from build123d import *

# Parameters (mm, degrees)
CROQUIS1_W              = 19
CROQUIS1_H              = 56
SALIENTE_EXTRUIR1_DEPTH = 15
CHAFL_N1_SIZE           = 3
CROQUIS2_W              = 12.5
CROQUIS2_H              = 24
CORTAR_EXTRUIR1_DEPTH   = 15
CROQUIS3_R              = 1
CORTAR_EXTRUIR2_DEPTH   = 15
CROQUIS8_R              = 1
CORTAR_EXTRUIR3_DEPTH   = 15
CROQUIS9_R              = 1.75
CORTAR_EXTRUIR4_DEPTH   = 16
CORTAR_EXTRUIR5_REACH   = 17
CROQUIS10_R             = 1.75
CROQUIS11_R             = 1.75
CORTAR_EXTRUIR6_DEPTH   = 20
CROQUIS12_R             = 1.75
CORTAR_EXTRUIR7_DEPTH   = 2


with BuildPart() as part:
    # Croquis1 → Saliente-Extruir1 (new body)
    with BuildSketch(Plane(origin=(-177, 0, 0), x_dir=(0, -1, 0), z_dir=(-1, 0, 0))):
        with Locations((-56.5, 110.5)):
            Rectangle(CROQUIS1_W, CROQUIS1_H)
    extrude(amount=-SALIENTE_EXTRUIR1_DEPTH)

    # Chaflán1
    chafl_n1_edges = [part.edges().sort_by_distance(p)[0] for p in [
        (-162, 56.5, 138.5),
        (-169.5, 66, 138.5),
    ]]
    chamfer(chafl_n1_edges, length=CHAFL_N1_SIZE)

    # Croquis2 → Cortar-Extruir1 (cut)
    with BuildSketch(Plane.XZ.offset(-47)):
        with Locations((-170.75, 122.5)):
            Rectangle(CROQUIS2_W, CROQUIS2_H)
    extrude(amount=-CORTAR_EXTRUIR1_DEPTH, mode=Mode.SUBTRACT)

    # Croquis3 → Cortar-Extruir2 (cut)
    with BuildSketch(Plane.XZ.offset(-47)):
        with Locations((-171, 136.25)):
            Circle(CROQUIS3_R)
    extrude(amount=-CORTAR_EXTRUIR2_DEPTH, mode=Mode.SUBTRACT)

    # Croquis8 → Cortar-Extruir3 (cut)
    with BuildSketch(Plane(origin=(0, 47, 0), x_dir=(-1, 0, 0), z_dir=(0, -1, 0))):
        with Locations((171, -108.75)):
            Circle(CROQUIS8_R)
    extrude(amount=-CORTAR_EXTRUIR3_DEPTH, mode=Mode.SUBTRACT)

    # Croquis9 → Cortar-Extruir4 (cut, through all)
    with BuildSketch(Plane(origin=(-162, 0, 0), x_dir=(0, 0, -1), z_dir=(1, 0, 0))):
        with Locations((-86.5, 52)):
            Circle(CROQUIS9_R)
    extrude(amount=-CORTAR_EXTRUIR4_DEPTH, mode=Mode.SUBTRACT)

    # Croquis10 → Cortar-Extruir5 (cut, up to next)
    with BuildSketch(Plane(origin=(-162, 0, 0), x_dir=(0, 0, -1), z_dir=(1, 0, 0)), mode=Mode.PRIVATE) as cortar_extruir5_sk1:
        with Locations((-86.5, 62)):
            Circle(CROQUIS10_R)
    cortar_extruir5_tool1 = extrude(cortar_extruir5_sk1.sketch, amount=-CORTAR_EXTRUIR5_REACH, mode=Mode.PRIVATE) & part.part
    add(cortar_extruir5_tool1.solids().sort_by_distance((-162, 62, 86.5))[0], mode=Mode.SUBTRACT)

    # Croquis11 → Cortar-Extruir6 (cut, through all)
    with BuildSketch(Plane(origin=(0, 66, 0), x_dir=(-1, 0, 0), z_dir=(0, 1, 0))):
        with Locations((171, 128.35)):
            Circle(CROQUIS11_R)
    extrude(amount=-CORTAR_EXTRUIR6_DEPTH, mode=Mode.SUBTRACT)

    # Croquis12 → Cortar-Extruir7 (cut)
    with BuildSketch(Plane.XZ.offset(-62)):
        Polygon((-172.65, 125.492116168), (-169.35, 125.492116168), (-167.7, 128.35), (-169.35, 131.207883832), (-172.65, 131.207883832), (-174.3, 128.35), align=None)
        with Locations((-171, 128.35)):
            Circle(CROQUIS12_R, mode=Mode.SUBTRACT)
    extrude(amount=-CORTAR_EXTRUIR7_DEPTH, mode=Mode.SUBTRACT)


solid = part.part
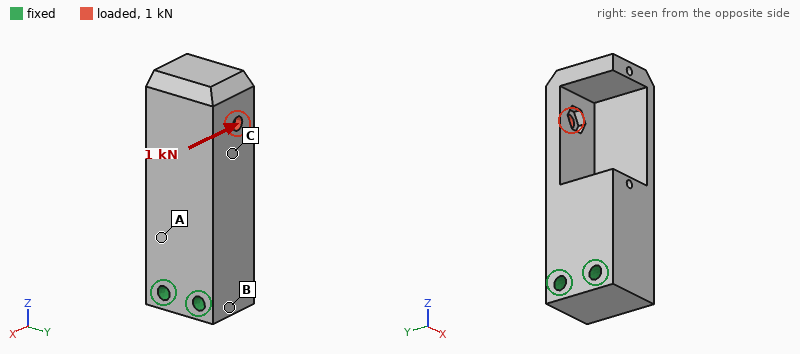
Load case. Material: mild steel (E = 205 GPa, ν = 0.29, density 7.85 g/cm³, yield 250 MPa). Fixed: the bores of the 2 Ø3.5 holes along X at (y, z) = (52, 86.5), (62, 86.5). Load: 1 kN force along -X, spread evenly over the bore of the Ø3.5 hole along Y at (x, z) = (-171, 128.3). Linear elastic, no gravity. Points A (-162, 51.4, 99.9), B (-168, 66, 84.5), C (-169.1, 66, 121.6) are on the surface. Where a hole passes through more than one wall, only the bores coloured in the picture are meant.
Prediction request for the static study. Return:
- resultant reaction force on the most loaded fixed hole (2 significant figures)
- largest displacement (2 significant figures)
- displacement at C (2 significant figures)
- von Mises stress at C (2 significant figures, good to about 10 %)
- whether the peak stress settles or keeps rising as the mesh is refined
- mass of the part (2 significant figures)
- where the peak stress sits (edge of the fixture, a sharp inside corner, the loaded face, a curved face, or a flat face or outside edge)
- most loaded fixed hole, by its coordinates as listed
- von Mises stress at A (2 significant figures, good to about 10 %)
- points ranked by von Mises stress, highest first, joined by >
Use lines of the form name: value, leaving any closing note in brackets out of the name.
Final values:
resultant reaction force on the most loaded fixed hole: 820 N
largest displacement: 61 µm
displacement at C: 30 µm
von Mises stress at C: 60 MPa
whether the peak stress settles or keeps rising as the mesh is refined: keeps rising
mass of the part: 85 g
where the peak stress sits: a sharp inside corner
most loaded fixed hole, by its coordinates as listed: (62, 86.5)
von Mises stress at A: 34 MPa
points ranked by von Mises stress, highest first, joined by >: C > A > B
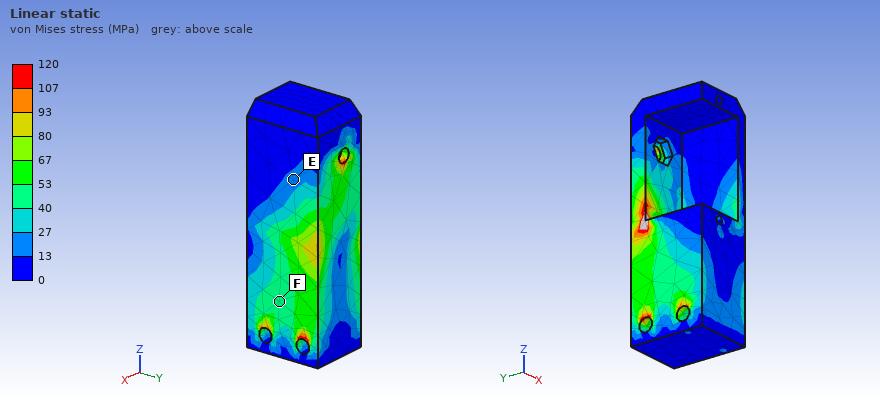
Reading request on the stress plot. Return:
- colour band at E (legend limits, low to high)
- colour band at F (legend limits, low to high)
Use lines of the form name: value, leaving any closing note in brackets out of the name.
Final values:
colour band at E: 13 to 27 MPa
colour band at F: 40 to 53 MPa
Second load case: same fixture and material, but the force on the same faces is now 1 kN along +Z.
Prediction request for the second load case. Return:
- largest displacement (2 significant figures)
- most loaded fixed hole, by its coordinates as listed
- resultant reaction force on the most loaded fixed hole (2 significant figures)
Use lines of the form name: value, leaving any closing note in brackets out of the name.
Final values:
largest displacement: 12 µm
most loaded fixed hole, by its coordinates as listed: (62, 86.5)
resultant reaction force on the most loaded fixed hole: 1.2 kN
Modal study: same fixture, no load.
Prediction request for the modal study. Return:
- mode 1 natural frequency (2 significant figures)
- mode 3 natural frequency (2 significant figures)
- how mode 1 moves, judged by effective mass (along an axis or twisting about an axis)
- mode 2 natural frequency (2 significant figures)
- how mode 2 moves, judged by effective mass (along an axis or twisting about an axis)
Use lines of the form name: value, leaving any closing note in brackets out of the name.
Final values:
mode 1 natural frequency: 4100 Hz
mode 3 natural frequency: 9300 Hz
how mode 1 moves, judged by effective mass: along X
mode 2 natural frequency: 5000 Hz
how mode 2 moves, judged by effective mass: along Y
